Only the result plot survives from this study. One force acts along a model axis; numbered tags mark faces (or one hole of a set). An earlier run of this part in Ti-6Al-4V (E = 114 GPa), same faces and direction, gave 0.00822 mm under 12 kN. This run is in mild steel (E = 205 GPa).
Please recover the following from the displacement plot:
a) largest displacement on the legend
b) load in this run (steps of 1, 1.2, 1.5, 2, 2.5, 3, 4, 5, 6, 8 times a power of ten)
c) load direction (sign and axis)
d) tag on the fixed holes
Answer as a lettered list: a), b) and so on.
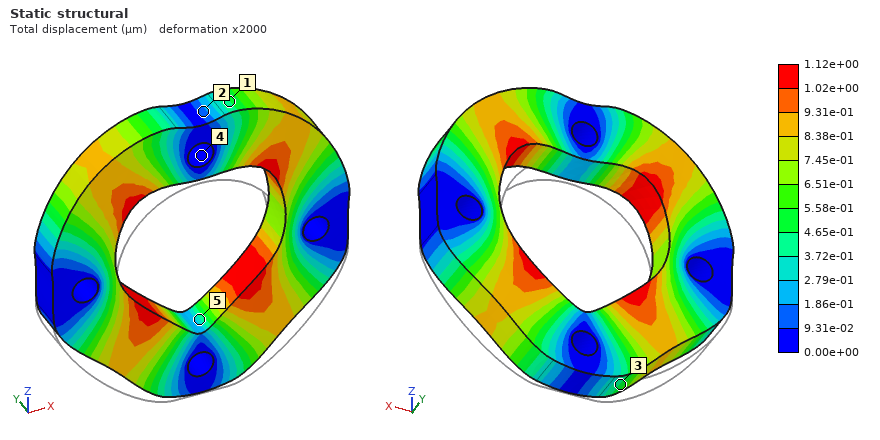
a) 1.12e+00 µm
b) 3 kN
c) +Z
d) 4
